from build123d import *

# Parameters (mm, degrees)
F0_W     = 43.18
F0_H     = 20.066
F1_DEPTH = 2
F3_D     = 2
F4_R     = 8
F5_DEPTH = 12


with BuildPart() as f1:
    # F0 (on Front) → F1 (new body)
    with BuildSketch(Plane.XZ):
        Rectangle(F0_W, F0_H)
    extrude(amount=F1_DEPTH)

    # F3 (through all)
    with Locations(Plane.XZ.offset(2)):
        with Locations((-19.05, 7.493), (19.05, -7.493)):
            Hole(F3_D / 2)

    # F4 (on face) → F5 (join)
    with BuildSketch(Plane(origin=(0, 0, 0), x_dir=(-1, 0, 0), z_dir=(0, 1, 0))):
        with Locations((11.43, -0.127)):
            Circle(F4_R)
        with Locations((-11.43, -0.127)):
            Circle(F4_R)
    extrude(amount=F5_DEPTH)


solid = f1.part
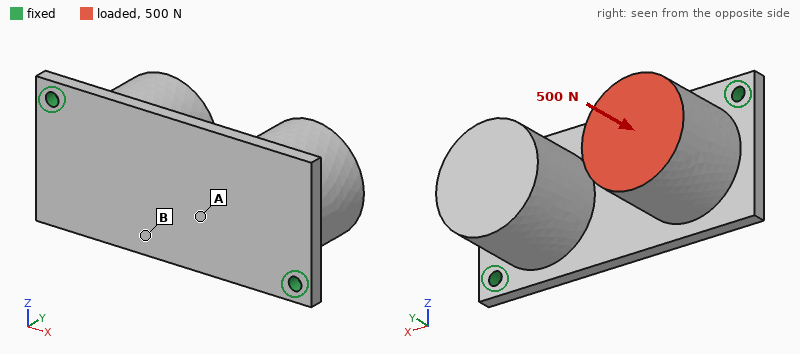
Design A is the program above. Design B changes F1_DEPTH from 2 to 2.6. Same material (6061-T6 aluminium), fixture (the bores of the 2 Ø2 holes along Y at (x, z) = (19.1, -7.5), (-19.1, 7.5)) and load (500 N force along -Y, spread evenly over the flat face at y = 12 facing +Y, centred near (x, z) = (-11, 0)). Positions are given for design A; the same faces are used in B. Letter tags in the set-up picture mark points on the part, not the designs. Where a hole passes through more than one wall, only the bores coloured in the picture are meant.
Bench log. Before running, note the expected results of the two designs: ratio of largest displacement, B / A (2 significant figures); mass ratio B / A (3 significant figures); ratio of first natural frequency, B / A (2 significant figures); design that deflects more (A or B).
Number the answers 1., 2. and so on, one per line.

1. 0.54
2. 1.08
3. 1.3
4. A
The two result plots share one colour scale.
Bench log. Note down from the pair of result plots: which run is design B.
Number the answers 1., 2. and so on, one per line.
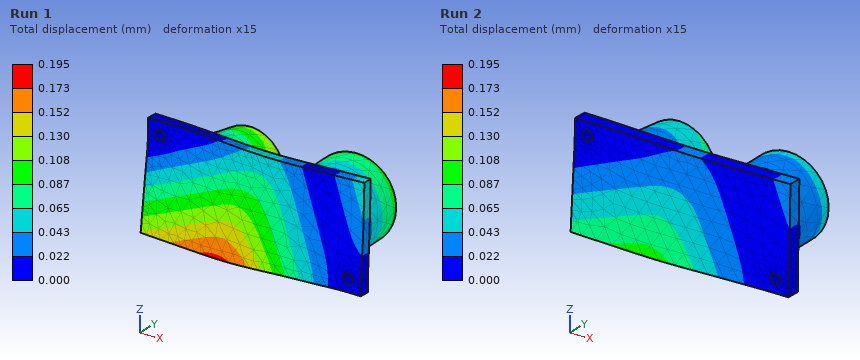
1. Run 2
